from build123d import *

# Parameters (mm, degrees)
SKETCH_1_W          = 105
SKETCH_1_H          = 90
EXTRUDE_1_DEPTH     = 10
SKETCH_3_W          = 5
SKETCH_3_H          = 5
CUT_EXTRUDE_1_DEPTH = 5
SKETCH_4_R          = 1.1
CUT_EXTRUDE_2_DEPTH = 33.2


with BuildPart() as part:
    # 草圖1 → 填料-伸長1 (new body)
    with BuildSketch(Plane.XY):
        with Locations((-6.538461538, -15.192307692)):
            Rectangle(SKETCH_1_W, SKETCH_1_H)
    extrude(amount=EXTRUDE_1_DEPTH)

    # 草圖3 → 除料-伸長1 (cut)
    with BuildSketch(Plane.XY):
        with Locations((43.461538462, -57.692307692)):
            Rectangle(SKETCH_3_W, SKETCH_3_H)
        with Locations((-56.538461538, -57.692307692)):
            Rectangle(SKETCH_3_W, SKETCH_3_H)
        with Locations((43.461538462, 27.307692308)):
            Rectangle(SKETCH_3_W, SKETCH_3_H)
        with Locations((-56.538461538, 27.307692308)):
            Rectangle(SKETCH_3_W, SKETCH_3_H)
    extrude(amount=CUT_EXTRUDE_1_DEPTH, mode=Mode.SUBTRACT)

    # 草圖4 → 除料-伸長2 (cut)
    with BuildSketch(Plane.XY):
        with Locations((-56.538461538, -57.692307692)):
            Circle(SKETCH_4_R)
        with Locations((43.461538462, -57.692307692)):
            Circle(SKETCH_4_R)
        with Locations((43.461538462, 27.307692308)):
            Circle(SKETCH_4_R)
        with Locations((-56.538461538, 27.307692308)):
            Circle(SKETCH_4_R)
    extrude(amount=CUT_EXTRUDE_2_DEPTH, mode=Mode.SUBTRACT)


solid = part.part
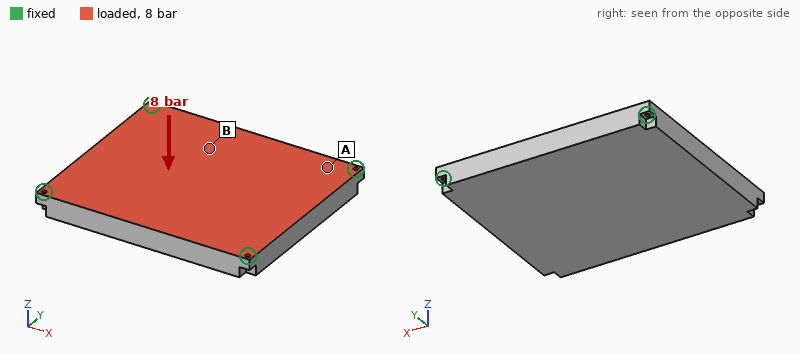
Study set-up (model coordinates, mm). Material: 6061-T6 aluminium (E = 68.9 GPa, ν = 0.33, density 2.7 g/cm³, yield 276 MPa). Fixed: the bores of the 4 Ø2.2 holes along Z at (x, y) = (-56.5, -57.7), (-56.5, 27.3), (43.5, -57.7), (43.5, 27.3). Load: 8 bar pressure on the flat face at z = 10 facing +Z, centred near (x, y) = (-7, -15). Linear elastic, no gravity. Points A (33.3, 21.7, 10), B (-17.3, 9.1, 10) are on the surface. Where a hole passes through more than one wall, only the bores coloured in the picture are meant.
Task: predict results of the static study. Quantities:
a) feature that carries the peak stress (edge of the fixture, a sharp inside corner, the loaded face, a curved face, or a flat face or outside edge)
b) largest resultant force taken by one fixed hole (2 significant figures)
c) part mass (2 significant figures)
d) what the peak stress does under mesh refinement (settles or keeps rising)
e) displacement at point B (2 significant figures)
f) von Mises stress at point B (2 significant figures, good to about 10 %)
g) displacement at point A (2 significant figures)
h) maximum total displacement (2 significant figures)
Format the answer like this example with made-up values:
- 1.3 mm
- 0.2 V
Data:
- edge of the fixture
- 3.1 kN
- 250 g
- keeps rising
- 0.15 mm
- 32 MPa
- 0.055 mm
- 0.17 mm
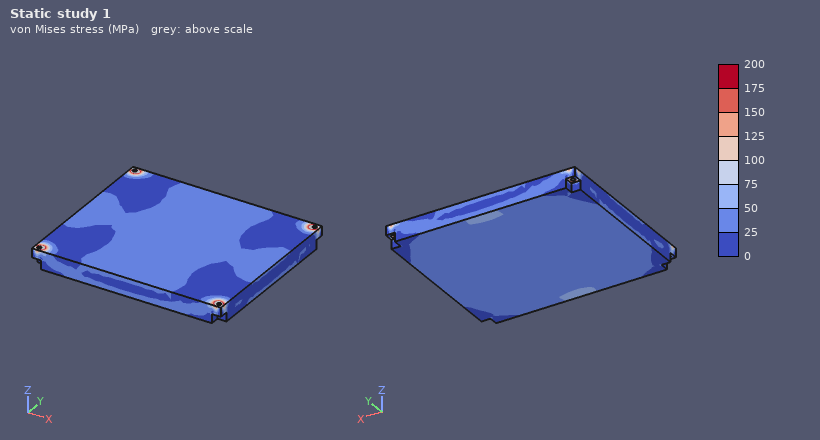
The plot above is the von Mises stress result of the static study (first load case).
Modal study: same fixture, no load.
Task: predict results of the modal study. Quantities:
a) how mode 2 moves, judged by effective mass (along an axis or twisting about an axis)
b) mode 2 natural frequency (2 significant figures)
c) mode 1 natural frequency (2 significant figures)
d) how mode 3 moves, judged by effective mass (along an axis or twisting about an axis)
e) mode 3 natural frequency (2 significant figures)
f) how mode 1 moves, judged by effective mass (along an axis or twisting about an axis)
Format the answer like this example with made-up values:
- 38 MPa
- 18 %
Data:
- twisting about X
- 4400 Hz
- 2400 Hz
- twisting about Y
- 4900 Hz
- along Z
